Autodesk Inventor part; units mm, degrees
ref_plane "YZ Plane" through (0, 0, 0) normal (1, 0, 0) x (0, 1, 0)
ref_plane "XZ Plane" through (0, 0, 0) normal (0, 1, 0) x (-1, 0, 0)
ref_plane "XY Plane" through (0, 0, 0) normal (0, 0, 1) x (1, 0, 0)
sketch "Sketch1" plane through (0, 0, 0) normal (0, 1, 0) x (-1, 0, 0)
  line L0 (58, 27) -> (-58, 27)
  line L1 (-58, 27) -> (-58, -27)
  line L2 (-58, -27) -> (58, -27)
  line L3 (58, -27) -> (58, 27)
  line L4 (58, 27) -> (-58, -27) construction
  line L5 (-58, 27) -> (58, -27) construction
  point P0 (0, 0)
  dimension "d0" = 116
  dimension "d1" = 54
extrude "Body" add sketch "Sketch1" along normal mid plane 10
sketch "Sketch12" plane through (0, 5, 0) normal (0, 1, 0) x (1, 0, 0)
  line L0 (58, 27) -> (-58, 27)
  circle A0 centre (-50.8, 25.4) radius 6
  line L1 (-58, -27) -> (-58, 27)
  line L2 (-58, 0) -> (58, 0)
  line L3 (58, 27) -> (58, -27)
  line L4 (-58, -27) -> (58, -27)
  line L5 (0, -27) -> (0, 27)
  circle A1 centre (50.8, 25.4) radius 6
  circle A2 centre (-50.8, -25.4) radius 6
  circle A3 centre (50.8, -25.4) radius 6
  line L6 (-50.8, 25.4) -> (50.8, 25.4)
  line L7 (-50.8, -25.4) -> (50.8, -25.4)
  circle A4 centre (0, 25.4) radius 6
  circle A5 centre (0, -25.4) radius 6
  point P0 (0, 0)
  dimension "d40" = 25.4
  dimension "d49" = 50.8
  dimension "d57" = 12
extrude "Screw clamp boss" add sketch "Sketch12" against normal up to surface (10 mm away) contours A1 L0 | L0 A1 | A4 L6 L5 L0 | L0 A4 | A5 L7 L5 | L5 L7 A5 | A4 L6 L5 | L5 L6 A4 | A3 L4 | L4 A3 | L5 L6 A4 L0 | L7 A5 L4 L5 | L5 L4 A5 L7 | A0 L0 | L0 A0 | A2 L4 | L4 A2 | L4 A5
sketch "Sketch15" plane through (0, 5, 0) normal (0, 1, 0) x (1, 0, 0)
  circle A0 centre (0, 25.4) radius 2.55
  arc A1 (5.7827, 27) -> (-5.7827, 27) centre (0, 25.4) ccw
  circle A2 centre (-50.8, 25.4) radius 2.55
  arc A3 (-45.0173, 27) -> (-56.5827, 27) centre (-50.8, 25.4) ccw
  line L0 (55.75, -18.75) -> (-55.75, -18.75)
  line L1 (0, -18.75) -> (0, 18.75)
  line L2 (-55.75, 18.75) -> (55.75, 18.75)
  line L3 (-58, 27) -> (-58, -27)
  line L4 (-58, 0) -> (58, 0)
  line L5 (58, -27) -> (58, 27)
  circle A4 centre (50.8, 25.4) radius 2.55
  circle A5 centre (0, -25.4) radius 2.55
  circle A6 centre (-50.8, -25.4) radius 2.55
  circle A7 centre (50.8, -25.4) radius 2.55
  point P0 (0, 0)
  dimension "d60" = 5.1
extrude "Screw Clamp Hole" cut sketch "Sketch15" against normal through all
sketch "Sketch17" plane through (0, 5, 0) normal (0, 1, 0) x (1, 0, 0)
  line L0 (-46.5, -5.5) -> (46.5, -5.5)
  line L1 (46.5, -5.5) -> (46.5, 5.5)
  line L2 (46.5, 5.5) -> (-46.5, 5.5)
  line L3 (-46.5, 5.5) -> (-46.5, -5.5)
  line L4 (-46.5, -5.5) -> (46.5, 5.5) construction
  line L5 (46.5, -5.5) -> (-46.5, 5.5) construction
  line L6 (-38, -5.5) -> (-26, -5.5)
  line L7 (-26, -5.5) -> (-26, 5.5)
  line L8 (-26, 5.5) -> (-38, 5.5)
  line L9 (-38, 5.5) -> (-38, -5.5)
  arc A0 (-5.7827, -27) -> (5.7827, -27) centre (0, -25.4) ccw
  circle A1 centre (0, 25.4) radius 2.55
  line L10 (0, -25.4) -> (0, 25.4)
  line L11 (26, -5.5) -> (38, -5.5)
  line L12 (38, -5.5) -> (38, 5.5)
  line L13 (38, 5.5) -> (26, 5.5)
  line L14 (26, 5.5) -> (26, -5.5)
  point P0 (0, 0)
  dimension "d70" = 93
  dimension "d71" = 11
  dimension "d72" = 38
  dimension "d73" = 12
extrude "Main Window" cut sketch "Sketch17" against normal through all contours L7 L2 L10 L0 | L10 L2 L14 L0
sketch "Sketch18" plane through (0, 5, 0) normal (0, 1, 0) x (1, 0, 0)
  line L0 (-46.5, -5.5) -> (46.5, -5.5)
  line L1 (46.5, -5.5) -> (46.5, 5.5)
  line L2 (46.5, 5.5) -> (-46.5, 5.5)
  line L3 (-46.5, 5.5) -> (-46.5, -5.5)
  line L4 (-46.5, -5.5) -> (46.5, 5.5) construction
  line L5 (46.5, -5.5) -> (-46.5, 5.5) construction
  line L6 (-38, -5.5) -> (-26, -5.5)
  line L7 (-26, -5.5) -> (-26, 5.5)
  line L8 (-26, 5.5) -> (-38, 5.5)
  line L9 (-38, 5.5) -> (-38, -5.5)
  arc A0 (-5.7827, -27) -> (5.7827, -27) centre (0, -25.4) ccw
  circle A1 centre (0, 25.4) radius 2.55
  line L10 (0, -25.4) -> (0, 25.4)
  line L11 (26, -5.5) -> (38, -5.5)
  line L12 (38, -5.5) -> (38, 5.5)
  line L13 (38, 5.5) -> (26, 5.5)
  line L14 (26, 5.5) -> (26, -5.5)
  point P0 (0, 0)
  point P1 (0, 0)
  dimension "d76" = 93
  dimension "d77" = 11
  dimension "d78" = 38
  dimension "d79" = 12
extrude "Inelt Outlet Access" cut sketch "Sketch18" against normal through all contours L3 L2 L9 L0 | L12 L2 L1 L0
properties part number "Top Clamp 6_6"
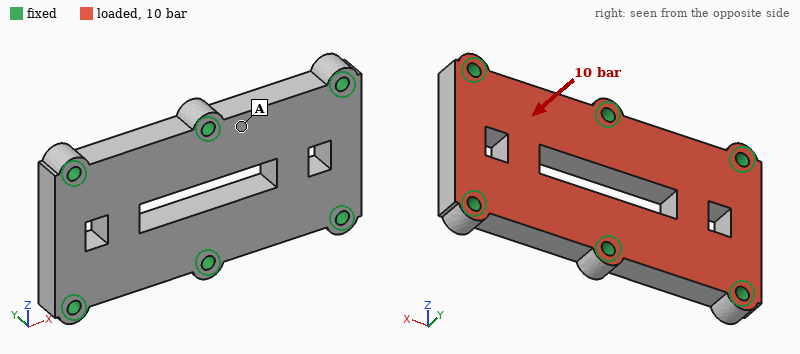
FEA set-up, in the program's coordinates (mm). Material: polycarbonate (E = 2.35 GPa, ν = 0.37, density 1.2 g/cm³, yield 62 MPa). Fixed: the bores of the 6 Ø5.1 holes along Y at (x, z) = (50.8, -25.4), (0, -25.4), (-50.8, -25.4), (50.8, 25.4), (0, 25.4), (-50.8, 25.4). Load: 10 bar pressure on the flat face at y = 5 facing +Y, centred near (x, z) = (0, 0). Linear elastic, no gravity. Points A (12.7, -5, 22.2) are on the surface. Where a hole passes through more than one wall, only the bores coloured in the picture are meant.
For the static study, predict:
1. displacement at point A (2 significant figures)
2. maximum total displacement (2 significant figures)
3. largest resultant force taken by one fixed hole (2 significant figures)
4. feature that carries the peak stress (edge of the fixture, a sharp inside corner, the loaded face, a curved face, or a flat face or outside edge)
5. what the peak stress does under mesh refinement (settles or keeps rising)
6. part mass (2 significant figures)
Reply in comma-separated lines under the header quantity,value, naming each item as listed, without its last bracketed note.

quantity,value
displacement at point A,0.12 mm
maximum total displacement,0.33 mm
largest resultant force taken by one fixed hole,1.2 kN
feature that carries the peak stress,edge of the fixture
what the peak stress does under mesh refinement,keeps rising
part mass,67 g
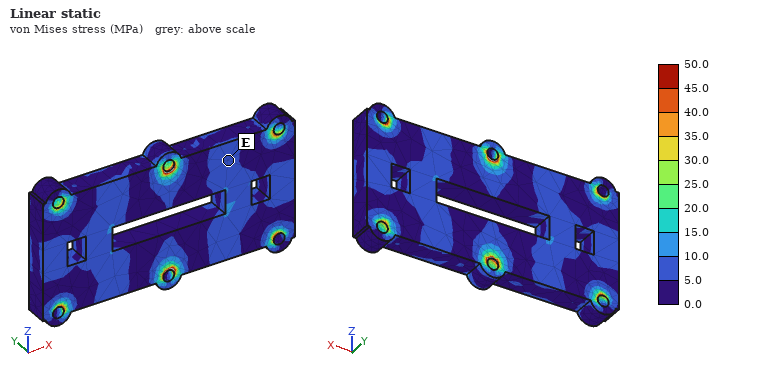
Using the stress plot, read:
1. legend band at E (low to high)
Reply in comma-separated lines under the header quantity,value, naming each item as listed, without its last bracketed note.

quantity,value
legend band at E,5.0 to 10.0 MPa
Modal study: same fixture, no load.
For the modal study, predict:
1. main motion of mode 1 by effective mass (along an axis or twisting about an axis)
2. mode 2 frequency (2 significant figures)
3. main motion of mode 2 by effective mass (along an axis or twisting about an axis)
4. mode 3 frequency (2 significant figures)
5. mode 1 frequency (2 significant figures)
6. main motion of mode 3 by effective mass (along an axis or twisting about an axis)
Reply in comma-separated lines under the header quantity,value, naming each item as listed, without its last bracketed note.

quantity,value
main motion of mode 1 by effective mass,along Y
mode 2 frequency,3300 Hz
main motion of mode 2 by effective mass,twisting about Z
mode 3 frequency,4600 Hz
mode 1 frequency,3100 Hz
main motion of mode 3 by effective mass,twisting about X
